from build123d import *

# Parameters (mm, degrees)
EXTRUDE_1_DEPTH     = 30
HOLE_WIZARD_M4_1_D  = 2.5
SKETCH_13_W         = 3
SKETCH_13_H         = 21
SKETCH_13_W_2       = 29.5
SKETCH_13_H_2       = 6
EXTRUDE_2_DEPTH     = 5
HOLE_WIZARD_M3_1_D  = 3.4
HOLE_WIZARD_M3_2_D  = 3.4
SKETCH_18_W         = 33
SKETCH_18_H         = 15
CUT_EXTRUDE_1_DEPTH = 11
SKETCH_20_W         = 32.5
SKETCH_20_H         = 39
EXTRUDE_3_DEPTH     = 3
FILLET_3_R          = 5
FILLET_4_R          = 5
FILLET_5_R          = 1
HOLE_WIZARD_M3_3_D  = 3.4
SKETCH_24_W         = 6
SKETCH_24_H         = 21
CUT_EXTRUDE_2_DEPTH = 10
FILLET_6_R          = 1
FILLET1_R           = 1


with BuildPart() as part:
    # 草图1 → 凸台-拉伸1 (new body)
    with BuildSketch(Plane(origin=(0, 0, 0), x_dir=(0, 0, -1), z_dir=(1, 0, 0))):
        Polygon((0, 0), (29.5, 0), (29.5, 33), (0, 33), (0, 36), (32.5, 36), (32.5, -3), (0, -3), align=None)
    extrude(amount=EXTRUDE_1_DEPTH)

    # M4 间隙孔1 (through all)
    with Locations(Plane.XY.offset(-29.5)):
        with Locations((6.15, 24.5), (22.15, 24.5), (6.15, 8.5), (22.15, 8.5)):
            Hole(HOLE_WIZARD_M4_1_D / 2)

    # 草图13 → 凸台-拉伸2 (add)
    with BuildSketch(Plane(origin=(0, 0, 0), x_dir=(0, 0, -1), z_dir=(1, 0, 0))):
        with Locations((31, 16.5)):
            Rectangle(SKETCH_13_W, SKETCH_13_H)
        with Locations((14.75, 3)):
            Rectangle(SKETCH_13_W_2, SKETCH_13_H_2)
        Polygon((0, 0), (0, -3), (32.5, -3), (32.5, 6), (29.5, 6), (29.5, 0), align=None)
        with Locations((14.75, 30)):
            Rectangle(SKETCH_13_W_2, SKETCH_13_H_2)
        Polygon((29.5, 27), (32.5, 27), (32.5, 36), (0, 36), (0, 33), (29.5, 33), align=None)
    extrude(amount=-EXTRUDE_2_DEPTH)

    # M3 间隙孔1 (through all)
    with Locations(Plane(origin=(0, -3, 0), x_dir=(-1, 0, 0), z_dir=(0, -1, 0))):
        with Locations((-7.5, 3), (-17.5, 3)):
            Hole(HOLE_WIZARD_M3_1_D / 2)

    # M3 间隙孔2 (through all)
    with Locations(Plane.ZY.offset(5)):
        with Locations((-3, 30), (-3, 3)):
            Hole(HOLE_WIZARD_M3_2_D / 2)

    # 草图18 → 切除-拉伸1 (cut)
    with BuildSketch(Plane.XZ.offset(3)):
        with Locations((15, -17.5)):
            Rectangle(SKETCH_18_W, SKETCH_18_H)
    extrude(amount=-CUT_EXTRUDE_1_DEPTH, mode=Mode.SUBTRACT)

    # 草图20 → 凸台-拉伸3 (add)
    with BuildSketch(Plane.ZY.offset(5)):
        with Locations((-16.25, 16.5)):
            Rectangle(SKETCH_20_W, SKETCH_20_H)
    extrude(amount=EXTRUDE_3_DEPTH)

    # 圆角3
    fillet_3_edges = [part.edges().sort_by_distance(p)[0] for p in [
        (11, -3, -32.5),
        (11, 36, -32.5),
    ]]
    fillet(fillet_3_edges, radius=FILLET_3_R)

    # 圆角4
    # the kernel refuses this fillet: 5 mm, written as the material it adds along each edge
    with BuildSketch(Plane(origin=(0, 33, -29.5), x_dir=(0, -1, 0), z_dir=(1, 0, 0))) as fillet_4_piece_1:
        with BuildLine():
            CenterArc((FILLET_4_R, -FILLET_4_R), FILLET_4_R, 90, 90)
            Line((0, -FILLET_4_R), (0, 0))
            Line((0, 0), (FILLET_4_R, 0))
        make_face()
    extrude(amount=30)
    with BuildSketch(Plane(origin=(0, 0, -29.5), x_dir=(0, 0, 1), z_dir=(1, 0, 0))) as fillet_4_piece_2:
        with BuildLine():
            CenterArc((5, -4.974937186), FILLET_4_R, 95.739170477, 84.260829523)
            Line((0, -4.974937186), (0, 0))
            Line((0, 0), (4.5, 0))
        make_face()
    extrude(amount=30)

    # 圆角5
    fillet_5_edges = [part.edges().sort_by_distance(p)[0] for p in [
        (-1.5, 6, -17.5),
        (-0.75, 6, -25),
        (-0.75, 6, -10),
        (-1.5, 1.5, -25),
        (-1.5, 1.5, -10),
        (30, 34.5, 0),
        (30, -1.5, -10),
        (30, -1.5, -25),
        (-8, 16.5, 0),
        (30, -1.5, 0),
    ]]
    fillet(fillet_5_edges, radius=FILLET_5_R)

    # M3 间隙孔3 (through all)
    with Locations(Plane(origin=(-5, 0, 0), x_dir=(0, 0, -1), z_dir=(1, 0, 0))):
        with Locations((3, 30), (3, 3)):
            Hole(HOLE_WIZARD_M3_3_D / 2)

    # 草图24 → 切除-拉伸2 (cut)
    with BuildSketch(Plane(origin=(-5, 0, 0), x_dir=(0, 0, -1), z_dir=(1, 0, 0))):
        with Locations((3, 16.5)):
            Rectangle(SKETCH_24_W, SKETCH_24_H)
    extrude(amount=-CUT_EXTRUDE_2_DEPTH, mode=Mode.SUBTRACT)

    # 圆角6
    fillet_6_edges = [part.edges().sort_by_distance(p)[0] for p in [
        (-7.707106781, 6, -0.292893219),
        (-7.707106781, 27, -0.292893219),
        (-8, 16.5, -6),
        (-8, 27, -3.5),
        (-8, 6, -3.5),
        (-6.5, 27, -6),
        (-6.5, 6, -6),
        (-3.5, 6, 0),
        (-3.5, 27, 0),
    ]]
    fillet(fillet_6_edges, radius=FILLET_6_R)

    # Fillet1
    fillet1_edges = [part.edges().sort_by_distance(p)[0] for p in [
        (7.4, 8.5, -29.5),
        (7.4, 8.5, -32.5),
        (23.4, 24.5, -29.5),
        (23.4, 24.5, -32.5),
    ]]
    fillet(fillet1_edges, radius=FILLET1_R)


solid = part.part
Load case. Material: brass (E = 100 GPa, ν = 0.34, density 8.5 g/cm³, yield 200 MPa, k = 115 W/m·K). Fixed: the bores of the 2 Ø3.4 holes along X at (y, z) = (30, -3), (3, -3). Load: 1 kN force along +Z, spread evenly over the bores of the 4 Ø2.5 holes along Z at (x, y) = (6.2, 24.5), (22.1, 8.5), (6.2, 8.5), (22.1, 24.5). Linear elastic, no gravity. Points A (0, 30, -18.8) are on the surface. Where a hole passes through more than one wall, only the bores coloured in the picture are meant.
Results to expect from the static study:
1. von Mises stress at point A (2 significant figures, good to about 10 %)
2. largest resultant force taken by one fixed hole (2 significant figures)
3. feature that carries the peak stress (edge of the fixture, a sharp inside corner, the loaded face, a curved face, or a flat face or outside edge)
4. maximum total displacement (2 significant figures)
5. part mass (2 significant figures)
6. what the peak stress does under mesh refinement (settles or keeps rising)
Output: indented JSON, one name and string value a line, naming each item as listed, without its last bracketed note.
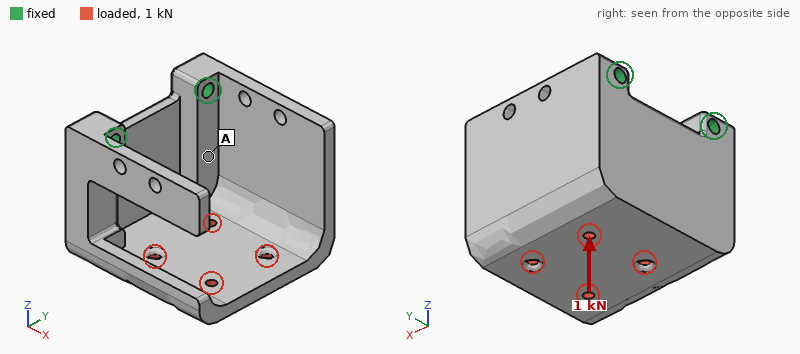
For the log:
{
  "von Mises stress at point A": "23 MPa",
  "largest resultant force taken by one fixed hole": "530 N",
  "feature that carries the peak stress": "edge of the fixture",
  "maximum total displacement": "0.27 mm",
  "part mass": "110 g",
  "what the peak stress does under mesh refinement": "keeps rising"
}
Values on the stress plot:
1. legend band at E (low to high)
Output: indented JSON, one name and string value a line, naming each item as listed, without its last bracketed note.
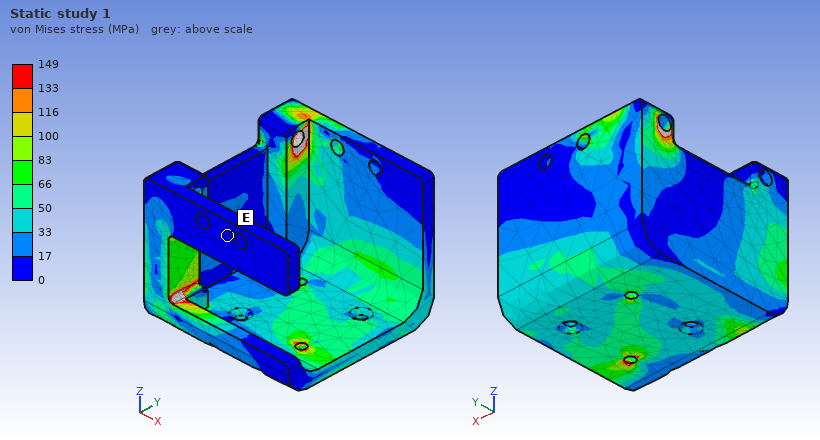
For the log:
{
  "legend band at E": "0 to 17 MPa"
}
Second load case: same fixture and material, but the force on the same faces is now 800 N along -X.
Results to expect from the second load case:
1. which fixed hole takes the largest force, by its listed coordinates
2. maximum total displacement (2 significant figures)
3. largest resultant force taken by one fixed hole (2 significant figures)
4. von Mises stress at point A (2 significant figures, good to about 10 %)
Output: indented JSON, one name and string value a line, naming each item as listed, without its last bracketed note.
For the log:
{
  "which fixed hole takes the largest force, by its listed coordinates": "(30, -3)",
  "maximum total displacement": "0.14 mm",
  "largest resultant force taken by one fixed hole": "460 N",
  "von Mises stress at point A": "15 MPa"
}
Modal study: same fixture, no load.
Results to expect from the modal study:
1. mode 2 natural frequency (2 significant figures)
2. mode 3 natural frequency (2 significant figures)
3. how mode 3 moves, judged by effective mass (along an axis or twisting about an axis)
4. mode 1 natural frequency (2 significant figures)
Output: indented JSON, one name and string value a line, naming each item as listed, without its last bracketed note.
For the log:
{
  "mode 2 natural frequency": "1700 Hz",
  "mode 3 natural frequency": "1900 Hz",
  "how mode 3 moves, judged by effective mass": "along Y",
  "mode 1 natural frequency": "1600 Hz"
}
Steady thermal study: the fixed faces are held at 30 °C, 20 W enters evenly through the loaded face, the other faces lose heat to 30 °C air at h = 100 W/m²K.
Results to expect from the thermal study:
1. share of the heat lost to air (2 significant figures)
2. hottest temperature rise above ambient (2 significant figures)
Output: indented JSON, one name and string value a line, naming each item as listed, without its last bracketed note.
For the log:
{
  "share of the heat lost to air": "48 %",
  "hottest temperature rise above ambient": "30 K"
}
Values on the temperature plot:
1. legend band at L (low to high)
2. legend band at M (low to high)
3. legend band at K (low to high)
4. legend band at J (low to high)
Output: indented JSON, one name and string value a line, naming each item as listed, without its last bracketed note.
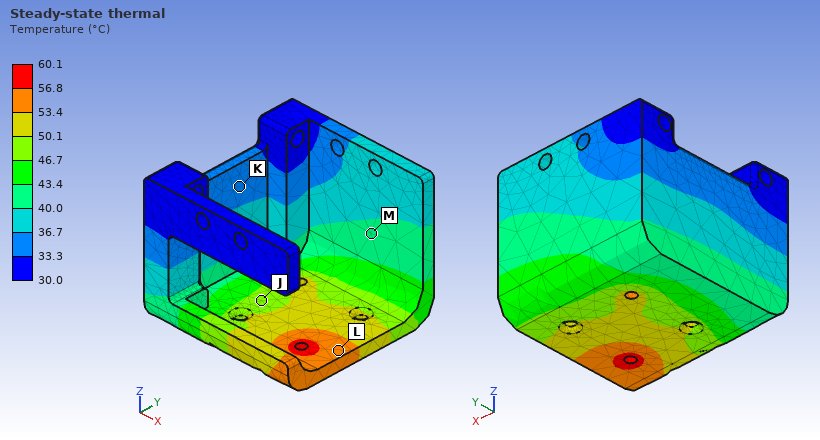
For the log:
{
  "legend band at L": "53.4 to 56.8 °C",
  "legend band at M": "40.0 to 43.4 °C",
  "legend band at K": "33.3 to 36.7 °C",
  "legend band at J": "46.7 to 50.1 °C"
}
